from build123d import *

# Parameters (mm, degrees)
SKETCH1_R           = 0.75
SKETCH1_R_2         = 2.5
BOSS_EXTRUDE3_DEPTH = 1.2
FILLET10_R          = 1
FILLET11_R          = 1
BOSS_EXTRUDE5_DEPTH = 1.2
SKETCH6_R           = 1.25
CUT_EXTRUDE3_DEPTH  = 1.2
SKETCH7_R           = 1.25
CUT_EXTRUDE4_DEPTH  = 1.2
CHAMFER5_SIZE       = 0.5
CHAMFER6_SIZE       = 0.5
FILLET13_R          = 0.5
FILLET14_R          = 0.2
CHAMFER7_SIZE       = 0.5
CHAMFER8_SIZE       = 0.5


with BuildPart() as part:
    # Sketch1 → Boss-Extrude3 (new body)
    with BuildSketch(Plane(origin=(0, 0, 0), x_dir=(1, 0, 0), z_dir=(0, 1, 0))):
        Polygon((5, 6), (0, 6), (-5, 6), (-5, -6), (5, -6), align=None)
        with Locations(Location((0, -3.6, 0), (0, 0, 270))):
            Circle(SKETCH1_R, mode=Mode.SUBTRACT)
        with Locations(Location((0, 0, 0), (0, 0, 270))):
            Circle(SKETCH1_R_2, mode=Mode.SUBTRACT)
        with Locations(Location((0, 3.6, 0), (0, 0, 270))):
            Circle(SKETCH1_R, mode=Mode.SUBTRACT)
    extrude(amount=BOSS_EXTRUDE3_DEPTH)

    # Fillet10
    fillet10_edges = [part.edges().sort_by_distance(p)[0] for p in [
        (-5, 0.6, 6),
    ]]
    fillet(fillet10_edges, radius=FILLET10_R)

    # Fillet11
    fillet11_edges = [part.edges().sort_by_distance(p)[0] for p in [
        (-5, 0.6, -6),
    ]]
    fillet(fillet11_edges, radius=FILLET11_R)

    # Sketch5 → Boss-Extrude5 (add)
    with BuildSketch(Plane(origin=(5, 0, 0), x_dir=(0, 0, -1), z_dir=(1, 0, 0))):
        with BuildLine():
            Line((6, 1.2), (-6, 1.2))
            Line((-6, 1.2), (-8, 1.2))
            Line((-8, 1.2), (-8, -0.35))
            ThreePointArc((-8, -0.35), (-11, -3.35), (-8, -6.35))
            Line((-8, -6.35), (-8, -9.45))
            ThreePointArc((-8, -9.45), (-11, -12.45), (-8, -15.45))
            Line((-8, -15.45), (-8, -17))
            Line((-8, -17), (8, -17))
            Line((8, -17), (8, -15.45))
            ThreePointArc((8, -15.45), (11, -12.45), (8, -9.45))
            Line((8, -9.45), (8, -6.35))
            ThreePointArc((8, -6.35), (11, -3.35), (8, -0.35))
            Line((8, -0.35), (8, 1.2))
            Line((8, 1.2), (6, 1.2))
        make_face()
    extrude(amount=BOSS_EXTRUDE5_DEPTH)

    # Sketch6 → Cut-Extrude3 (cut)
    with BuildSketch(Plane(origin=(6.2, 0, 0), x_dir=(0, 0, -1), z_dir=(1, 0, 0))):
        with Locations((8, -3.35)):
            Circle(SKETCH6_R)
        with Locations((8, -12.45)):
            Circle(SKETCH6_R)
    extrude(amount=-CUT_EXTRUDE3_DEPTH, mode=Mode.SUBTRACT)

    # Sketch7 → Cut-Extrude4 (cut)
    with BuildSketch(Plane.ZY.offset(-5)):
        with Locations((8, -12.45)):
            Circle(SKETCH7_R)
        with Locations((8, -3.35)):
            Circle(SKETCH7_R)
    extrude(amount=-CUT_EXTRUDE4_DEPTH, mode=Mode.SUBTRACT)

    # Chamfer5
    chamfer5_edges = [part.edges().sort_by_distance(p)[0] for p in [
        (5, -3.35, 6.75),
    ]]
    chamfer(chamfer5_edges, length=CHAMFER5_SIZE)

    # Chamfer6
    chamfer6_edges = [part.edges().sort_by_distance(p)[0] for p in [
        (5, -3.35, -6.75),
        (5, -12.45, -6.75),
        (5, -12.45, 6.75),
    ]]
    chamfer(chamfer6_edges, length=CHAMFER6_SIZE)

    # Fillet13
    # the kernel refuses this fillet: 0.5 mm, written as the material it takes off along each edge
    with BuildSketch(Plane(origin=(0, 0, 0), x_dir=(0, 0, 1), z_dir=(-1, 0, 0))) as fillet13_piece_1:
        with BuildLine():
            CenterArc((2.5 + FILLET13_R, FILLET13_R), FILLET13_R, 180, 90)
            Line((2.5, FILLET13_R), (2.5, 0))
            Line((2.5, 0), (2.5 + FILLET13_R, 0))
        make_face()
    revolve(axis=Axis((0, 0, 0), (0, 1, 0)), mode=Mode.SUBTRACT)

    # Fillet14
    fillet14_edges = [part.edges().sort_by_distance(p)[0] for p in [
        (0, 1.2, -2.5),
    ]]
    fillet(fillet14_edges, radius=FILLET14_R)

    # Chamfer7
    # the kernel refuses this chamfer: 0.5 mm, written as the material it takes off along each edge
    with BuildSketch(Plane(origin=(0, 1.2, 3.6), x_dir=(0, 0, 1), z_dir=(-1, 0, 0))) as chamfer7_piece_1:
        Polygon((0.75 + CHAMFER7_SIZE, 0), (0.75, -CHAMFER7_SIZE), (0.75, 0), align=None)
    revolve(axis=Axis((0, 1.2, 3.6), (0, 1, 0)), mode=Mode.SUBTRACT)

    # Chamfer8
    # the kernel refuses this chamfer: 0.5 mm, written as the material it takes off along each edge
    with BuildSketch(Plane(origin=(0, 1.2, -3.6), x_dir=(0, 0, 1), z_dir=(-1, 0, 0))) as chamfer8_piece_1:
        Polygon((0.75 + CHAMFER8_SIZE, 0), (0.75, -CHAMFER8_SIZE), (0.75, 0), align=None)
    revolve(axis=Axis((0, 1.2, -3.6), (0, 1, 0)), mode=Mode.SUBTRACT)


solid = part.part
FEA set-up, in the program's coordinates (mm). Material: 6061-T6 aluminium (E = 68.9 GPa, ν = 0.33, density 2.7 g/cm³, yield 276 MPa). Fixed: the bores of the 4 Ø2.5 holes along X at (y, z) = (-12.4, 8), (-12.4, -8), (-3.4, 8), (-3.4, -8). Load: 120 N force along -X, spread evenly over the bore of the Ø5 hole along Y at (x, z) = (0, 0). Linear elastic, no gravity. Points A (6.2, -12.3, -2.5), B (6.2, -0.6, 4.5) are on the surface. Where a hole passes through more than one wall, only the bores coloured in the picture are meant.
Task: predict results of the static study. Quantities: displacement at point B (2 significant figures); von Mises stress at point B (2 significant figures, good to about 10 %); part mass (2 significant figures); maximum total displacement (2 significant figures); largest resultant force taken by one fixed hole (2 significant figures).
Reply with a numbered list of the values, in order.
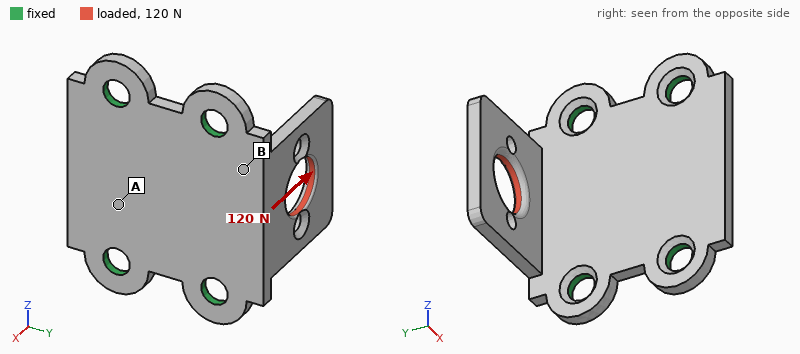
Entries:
1. 17 µm
2. 42 MPa
3. 1.4 g
4. 88 µm
5. 82 N
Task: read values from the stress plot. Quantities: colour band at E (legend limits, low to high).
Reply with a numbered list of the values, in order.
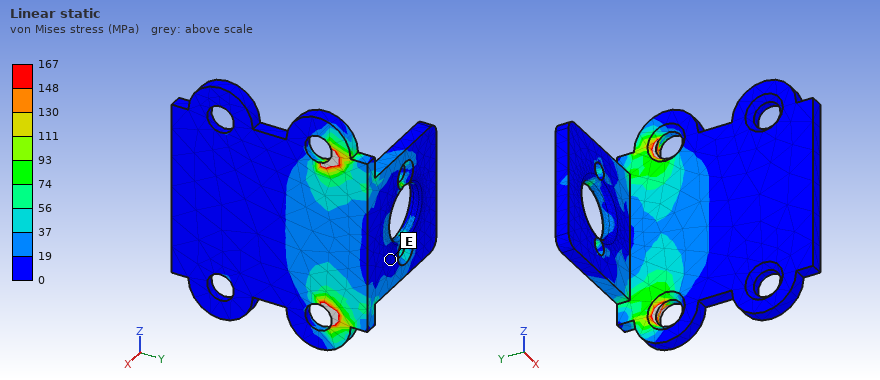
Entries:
1. 0 to 19 MPa
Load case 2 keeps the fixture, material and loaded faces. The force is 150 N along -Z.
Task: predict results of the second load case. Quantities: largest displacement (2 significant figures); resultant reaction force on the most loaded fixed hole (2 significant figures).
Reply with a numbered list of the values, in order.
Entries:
1. 43 µm
2. 100 N
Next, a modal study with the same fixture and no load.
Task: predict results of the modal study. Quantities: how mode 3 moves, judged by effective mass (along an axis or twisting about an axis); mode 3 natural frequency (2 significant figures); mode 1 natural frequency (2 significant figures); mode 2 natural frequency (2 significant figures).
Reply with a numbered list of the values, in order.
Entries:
1. along X
2. 19 kHz
3. 6000 Hz
4. 14 kHz
